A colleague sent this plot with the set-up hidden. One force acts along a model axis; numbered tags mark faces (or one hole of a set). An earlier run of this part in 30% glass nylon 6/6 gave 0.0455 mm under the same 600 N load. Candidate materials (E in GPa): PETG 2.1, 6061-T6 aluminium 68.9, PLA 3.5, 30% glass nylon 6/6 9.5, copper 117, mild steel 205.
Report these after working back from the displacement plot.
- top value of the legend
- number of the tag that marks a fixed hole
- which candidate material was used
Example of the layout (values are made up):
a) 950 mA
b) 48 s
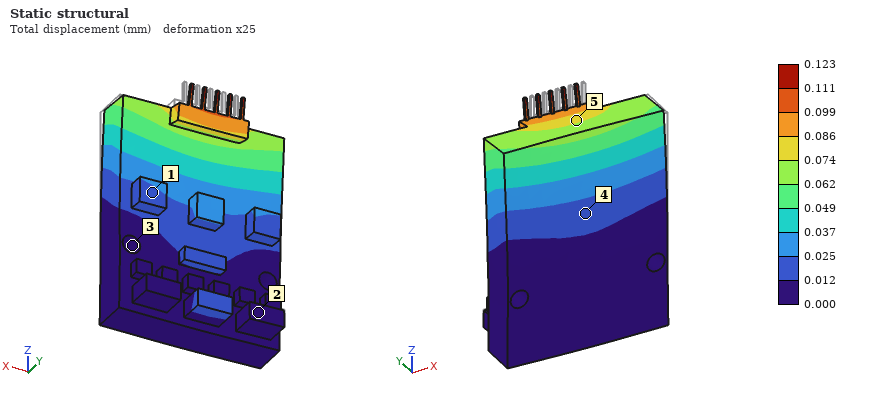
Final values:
a) 0.123 mm
b) 3
c) PLA
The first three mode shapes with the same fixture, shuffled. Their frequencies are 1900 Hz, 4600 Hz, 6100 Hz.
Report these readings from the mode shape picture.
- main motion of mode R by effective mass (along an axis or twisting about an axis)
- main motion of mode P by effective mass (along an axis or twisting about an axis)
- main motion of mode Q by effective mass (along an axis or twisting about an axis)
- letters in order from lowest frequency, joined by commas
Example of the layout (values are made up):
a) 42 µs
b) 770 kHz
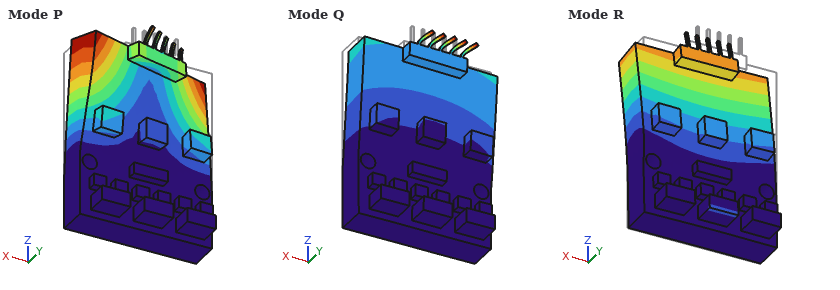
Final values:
a) along Y
b) twisting about Z
c) along X
d) R, P, Q
